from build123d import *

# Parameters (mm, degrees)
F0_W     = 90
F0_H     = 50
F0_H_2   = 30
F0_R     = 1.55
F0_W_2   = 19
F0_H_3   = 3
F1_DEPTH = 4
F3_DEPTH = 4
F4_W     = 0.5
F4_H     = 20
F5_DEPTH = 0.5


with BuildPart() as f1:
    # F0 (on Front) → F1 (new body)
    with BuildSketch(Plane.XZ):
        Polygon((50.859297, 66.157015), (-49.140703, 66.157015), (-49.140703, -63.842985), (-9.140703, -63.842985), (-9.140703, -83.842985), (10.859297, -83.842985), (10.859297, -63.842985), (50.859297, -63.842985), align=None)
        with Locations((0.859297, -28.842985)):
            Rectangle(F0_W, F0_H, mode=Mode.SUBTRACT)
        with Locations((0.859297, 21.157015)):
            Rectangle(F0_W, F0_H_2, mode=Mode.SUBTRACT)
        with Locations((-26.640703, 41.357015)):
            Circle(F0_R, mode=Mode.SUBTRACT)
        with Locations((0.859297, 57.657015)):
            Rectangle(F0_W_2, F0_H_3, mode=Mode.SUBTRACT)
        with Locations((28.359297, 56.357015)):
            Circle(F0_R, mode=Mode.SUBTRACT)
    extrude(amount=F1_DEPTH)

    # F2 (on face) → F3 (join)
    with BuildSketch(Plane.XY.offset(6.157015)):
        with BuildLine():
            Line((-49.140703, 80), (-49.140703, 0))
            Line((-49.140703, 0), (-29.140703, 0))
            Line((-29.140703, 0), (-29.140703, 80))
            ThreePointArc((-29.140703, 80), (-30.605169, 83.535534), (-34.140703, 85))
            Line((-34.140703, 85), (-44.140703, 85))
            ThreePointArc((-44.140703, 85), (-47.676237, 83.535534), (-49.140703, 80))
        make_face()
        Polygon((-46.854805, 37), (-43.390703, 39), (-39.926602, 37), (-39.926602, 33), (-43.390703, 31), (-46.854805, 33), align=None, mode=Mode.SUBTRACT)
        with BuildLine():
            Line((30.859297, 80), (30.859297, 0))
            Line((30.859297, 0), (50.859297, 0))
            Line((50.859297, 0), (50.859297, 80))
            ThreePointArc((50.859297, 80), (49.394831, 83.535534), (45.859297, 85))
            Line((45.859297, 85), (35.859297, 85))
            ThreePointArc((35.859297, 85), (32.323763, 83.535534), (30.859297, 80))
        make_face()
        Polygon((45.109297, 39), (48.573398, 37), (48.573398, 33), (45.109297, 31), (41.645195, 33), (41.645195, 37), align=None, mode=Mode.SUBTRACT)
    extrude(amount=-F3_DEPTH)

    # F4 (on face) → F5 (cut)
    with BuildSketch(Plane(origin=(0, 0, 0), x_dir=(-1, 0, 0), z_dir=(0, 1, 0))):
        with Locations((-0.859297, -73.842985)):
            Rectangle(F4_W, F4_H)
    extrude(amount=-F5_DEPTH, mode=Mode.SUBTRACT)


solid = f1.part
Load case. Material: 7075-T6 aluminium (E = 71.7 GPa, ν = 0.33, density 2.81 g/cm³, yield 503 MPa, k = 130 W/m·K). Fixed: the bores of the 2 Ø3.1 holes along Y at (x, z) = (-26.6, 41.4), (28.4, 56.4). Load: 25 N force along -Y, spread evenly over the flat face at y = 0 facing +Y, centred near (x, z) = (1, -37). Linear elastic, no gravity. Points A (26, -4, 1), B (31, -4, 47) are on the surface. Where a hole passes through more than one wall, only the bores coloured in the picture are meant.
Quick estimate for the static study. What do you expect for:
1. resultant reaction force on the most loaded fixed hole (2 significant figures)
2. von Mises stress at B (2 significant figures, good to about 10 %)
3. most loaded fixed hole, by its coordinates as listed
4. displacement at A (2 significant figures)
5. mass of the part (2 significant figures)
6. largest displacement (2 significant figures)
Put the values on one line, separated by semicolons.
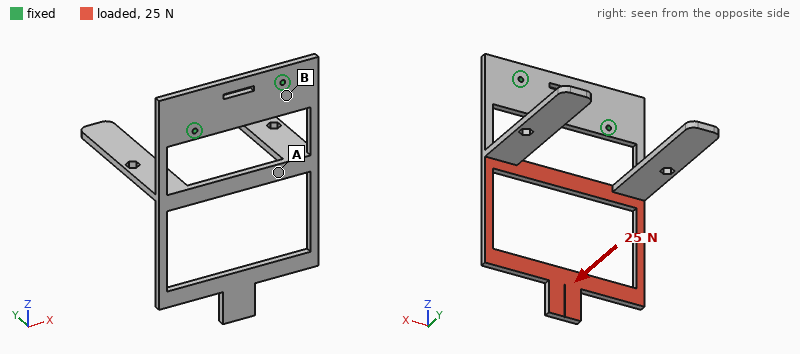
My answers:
16 N; 11 MPa; (28.4, 56.4); 0.44 mm; 110 g; 2.3 mm
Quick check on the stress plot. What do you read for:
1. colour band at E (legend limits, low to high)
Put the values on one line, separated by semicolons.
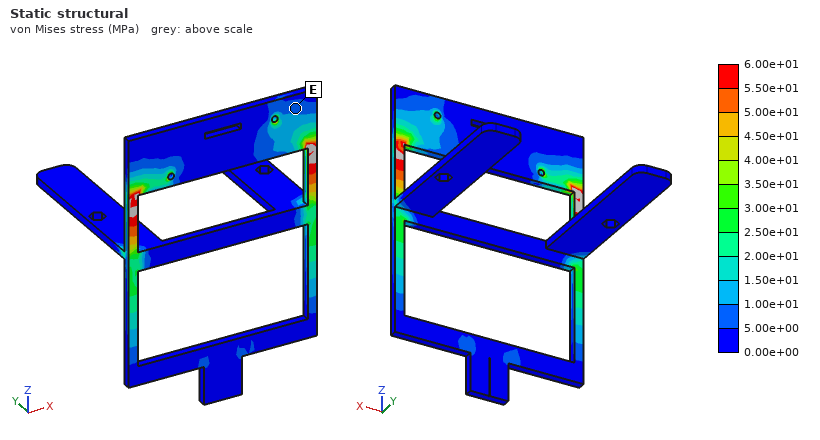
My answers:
5.00e+00 to 1.00e+01 MPa
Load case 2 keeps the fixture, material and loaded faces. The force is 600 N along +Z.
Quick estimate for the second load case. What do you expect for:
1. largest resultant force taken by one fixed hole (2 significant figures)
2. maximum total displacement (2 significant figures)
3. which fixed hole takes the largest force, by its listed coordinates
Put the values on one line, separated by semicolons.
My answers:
330 N; 2.0 mm; (28.4, 56.4)
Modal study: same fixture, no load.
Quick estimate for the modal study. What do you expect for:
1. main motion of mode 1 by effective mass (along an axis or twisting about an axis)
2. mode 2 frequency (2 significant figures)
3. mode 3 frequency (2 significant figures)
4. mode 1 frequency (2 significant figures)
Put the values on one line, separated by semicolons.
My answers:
along Y; 230 Hz; 290 Hz; 92 Hz
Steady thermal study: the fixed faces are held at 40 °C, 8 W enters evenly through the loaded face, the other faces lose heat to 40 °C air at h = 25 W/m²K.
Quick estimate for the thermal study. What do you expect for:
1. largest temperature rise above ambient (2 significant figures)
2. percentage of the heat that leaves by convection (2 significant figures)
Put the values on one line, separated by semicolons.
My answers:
41 K; 80 %
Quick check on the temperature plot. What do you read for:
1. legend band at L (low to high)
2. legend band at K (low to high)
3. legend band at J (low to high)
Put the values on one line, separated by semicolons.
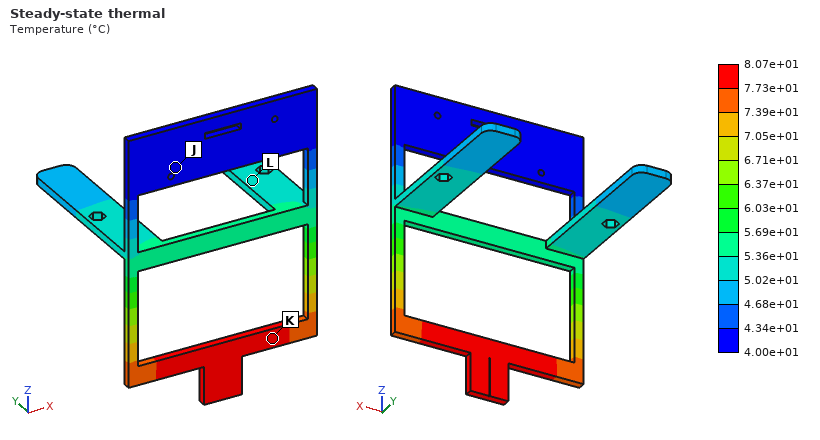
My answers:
5.02e+01 to 5.36e+01 °C; 7.73e+01 to 8.07e+01 °C; 4.00e+01 to 4.34e+01 °C
